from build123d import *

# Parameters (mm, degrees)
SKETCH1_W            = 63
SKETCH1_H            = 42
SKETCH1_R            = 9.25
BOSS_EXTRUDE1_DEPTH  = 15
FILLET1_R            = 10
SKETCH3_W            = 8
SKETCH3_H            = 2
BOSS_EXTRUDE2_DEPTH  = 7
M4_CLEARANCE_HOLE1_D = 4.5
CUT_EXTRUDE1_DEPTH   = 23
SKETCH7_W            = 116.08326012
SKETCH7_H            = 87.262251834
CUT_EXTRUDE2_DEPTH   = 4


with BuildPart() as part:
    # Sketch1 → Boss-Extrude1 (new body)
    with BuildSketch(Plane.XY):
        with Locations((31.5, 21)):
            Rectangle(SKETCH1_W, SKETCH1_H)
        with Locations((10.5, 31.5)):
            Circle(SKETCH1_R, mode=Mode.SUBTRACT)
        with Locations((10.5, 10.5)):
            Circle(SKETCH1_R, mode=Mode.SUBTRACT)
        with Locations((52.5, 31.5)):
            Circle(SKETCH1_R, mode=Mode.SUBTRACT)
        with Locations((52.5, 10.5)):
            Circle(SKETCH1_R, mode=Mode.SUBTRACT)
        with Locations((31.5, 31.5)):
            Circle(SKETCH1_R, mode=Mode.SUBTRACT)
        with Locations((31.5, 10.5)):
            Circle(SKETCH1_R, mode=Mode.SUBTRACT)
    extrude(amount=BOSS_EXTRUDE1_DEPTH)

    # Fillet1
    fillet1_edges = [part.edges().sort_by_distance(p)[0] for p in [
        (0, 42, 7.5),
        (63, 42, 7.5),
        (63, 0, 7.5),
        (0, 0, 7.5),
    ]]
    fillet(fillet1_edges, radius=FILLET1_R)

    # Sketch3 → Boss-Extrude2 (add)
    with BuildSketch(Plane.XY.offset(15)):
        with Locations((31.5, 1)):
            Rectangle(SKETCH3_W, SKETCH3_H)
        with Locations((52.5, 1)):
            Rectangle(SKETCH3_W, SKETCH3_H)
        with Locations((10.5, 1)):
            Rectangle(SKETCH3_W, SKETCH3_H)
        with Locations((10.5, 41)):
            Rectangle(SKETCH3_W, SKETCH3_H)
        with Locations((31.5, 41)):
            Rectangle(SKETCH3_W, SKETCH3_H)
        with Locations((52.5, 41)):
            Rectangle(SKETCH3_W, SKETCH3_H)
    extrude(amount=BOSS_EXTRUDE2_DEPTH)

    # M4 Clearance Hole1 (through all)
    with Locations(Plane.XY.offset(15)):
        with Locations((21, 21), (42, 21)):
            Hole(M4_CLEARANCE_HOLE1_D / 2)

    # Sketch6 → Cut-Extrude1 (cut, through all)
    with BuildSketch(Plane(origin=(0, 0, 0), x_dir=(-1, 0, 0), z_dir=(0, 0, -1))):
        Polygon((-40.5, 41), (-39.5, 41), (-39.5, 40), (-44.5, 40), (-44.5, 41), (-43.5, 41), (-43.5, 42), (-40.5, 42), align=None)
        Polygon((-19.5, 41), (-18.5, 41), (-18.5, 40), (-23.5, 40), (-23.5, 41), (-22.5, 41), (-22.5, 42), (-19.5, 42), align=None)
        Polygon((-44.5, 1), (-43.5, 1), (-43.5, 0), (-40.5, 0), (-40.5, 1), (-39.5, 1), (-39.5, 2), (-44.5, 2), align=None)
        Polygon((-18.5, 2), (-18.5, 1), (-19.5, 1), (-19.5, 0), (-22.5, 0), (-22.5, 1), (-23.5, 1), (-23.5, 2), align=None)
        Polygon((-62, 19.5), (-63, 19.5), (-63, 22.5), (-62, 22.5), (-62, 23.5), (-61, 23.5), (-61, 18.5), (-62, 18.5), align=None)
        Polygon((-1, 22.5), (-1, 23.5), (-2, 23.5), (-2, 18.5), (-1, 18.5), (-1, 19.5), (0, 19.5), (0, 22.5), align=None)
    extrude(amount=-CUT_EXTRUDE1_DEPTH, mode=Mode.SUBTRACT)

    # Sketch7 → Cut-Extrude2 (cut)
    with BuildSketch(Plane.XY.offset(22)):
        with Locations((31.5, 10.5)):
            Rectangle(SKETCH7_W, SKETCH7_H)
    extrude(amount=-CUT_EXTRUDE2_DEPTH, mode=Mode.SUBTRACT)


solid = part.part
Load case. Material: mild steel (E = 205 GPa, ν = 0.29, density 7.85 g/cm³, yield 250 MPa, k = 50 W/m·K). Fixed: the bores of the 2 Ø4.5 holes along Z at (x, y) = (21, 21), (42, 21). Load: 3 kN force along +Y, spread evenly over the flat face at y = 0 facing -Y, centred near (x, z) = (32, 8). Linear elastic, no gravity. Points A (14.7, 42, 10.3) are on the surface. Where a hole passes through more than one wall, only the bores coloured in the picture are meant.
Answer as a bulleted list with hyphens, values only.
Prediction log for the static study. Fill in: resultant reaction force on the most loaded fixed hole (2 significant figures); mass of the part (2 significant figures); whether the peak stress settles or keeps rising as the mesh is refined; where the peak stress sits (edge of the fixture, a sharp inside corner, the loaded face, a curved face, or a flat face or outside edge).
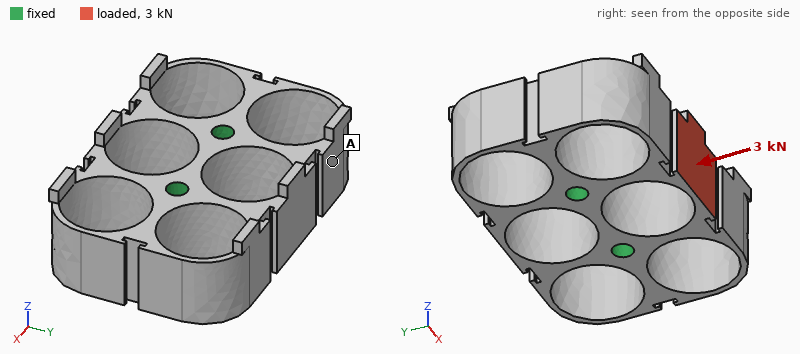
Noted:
- 1.7 kN
- 100 g
- keeps rising
- a sharp inside corner
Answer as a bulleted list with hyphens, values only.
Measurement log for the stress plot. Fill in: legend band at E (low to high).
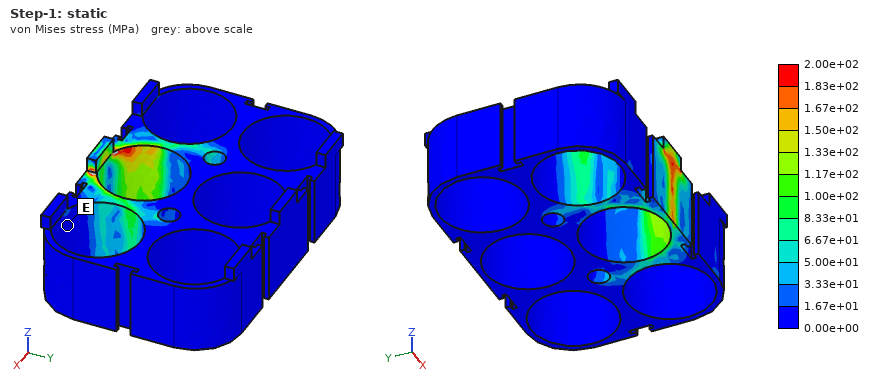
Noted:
- 0.00e+00 to 1.67e+01 MPa
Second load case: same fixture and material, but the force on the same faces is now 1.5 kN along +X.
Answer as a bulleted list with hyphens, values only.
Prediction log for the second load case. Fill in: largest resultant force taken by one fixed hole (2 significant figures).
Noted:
- 1.0 kN
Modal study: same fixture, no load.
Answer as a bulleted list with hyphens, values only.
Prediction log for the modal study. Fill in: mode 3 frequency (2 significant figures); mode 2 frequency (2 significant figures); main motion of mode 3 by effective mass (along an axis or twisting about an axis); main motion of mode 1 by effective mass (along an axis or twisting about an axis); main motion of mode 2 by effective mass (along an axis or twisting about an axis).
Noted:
- 9100 Hz
- 7800 Hz
- along X
- twisting about Z
- along Y
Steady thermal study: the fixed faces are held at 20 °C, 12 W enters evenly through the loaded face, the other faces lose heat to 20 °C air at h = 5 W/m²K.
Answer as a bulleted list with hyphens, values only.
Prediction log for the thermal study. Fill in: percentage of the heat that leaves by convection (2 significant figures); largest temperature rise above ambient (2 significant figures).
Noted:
- 3.5 %
- 51 K
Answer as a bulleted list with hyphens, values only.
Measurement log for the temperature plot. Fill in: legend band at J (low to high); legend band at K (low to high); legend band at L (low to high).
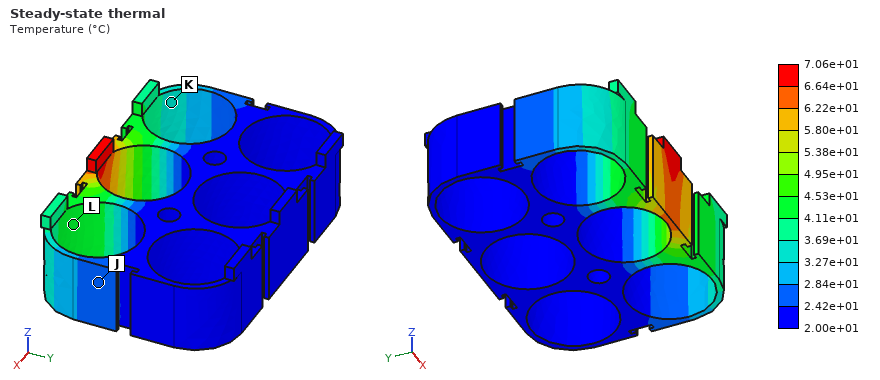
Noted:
- 2.42e+01 to 2.84e+01 °C
- 3.27e+01 to 3.69e+01 °C
- 4.11e+01 to 4.53e+01 °C
